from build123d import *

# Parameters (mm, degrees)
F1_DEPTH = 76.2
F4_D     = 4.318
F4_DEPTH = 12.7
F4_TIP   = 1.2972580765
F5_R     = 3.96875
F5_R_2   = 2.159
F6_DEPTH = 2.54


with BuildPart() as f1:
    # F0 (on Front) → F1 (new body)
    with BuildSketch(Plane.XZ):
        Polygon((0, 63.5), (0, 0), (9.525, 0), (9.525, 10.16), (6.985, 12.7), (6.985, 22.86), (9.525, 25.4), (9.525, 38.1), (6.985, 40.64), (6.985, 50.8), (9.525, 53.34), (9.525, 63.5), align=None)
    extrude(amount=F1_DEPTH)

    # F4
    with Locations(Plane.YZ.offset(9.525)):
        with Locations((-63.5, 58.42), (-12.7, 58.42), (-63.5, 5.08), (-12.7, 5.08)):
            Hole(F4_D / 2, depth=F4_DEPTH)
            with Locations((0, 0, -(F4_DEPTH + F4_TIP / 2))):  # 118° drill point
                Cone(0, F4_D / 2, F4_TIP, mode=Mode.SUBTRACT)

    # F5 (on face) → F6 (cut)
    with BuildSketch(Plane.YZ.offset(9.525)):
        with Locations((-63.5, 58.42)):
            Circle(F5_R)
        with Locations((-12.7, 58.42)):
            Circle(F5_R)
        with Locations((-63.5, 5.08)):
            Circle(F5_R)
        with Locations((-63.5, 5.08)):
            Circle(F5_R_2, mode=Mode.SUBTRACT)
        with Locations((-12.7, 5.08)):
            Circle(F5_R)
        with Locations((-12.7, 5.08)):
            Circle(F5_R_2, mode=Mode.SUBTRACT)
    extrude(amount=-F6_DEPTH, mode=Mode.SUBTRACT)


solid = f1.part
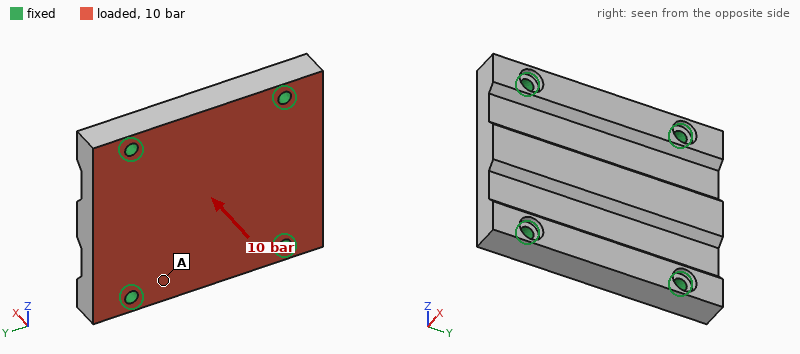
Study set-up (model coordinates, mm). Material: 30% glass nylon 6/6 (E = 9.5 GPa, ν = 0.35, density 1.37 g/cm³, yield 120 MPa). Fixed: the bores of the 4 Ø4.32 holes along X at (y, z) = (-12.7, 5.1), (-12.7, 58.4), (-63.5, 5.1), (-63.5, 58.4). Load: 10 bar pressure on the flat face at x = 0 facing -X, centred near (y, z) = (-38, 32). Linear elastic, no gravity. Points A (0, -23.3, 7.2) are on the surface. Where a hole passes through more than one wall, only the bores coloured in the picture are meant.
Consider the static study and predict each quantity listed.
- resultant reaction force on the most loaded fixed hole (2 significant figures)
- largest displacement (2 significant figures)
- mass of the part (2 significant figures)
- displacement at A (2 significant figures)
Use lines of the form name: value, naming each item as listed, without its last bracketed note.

resultant reaction force on the most loaded fixed hole: 1.2 kN
largest displacement: 0.14 mm
mass of the part: 55 g
displacement at A: 0.052 mm
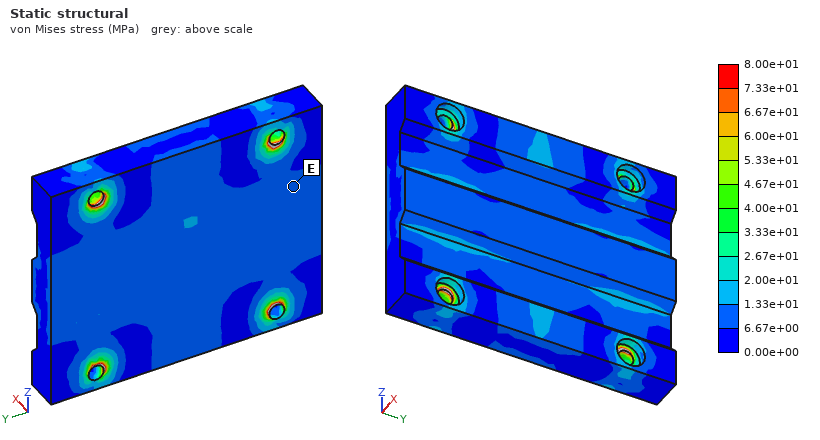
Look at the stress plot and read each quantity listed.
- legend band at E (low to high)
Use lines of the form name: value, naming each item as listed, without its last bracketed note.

legend band at E: 6.67e+00 to 1.33e+01 MPa
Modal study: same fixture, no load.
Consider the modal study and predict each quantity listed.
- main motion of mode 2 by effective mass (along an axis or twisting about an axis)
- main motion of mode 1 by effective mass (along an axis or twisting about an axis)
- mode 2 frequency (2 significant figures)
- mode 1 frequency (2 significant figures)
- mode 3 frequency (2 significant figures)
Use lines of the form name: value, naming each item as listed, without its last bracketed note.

main motion of mode 2 by effective mass: twisting about Z
main motion of mode 1 by effective mass: along X
mode 2 frequency: 6000 Hz
mode 1 frequency: 4600 Hz
mode 3 frequency: 6500 Hz
